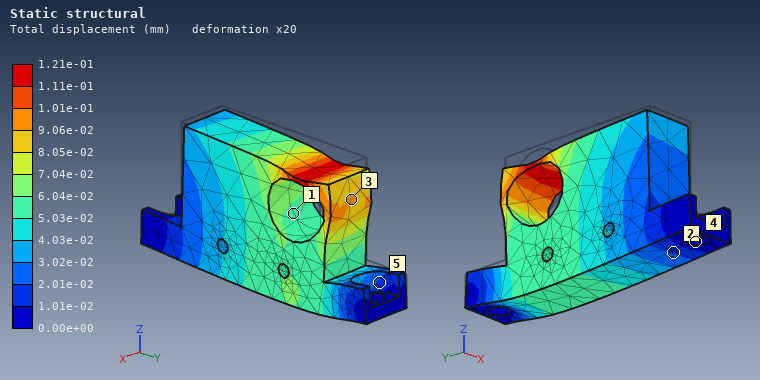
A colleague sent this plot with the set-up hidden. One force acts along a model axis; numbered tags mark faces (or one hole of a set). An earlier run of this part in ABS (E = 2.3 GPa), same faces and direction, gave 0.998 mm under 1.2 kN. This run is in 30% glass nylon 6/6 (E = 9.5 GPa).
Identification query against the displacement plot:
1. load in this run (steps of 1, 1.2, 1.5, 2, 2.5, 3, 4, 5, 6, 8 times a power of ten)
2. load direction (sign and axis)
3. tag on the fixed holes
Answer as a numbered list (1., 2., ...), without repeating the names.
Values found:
1. 600 N
2. -Z
3. 4
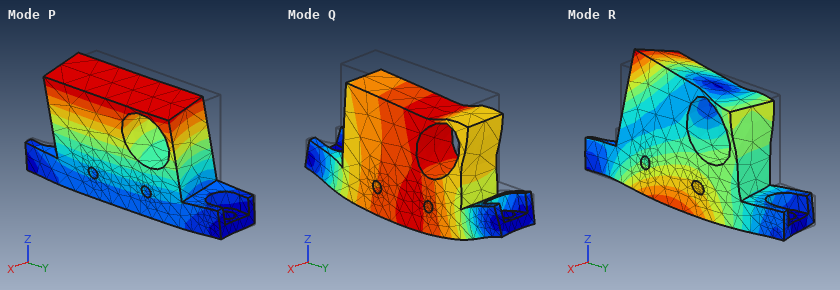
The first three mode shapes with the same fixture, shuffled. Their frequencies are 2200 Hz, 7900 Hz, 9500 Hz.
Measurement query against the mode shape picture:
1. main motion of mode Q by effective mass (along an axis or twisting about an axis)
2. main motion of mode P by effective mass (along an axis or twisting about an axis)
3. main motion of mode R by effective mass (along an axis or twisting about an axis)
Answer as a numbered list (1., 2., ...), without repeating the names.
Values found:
1. along Z
2. along X
3. along X
